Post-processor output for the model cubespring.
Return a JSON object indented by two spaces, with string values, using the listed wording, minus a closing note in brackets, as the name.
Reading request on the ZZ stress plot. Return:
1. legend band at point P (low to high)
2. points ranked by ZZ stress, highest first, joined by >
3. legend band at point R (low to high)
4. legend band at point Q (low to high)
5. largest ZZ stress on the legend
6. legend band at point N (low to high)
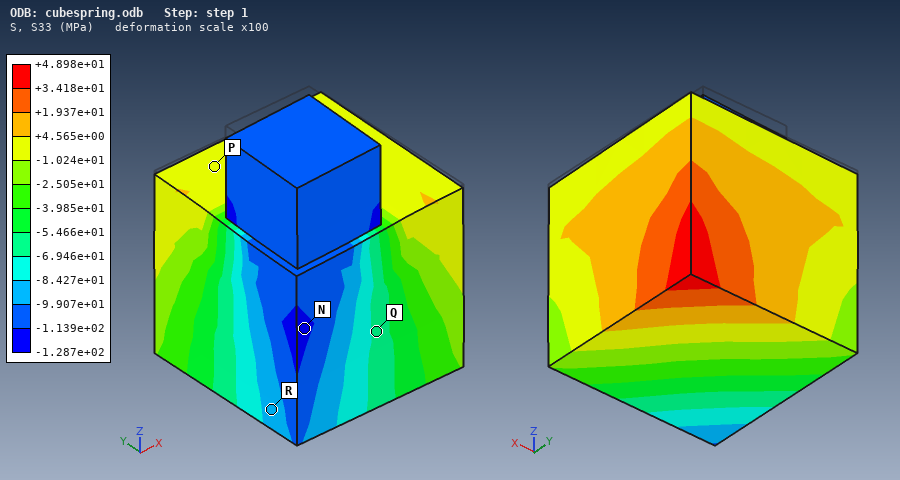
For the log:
{
  "legend band at point P": "-1.024e+01 to +4.565e+00 MPa",
  "points ranked by ZZ stress, highest first, joined by >": "P > Q > R > N",
  "legend band at point R": "-9.907e+01 to -8.427e+01 MPa",
  "legend band at point Q": "-6.946e+01 to -5.466e+01 MPa",
  "largest ZZ stress on the legend": "+4.898e+01 MPa",
  "legend band at point N": "-1.287e+02 to -1.139e+02 MPa"
}
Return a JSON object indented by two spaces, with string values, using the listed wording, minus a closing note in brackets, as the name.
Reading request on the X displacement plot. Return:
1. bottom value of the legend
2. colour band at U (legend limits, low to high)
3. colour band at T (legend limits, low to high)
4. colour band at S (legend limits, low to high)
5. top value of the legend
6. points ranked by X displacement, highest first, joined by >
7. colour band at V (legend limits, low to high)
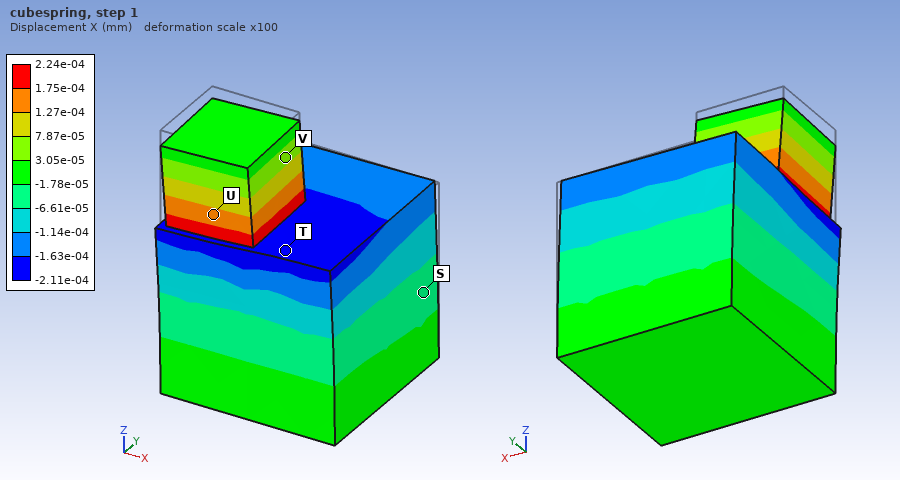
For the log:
{
  "bottom value of the legend": "-2.11e-04 mm",
  "colour band at U": "1.27e-04 to 1.75e-04 mm",
  "colour band at T": "-2.11e-04 to -1.63e-04 mm",
  "colour band at S": "-6.61e-05 to -1.78e-05 mm",
  "top value of the legend": "2.24e-04 mm",
  "points ranked by X displacement, highest first, joined by >": "U > V > S > T",
  "colour band at V": "3.05e-05 to 7.87e-05 mm"
}
